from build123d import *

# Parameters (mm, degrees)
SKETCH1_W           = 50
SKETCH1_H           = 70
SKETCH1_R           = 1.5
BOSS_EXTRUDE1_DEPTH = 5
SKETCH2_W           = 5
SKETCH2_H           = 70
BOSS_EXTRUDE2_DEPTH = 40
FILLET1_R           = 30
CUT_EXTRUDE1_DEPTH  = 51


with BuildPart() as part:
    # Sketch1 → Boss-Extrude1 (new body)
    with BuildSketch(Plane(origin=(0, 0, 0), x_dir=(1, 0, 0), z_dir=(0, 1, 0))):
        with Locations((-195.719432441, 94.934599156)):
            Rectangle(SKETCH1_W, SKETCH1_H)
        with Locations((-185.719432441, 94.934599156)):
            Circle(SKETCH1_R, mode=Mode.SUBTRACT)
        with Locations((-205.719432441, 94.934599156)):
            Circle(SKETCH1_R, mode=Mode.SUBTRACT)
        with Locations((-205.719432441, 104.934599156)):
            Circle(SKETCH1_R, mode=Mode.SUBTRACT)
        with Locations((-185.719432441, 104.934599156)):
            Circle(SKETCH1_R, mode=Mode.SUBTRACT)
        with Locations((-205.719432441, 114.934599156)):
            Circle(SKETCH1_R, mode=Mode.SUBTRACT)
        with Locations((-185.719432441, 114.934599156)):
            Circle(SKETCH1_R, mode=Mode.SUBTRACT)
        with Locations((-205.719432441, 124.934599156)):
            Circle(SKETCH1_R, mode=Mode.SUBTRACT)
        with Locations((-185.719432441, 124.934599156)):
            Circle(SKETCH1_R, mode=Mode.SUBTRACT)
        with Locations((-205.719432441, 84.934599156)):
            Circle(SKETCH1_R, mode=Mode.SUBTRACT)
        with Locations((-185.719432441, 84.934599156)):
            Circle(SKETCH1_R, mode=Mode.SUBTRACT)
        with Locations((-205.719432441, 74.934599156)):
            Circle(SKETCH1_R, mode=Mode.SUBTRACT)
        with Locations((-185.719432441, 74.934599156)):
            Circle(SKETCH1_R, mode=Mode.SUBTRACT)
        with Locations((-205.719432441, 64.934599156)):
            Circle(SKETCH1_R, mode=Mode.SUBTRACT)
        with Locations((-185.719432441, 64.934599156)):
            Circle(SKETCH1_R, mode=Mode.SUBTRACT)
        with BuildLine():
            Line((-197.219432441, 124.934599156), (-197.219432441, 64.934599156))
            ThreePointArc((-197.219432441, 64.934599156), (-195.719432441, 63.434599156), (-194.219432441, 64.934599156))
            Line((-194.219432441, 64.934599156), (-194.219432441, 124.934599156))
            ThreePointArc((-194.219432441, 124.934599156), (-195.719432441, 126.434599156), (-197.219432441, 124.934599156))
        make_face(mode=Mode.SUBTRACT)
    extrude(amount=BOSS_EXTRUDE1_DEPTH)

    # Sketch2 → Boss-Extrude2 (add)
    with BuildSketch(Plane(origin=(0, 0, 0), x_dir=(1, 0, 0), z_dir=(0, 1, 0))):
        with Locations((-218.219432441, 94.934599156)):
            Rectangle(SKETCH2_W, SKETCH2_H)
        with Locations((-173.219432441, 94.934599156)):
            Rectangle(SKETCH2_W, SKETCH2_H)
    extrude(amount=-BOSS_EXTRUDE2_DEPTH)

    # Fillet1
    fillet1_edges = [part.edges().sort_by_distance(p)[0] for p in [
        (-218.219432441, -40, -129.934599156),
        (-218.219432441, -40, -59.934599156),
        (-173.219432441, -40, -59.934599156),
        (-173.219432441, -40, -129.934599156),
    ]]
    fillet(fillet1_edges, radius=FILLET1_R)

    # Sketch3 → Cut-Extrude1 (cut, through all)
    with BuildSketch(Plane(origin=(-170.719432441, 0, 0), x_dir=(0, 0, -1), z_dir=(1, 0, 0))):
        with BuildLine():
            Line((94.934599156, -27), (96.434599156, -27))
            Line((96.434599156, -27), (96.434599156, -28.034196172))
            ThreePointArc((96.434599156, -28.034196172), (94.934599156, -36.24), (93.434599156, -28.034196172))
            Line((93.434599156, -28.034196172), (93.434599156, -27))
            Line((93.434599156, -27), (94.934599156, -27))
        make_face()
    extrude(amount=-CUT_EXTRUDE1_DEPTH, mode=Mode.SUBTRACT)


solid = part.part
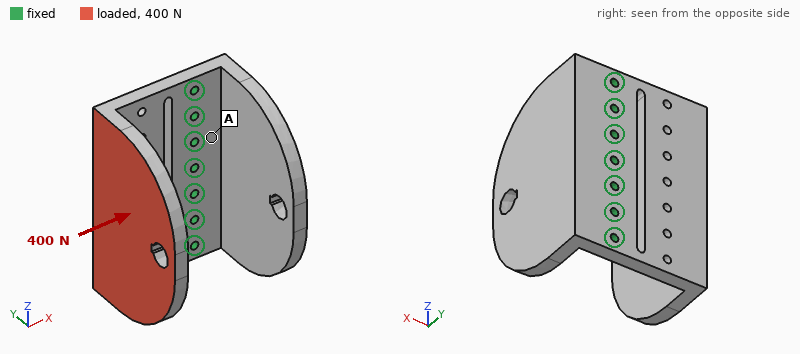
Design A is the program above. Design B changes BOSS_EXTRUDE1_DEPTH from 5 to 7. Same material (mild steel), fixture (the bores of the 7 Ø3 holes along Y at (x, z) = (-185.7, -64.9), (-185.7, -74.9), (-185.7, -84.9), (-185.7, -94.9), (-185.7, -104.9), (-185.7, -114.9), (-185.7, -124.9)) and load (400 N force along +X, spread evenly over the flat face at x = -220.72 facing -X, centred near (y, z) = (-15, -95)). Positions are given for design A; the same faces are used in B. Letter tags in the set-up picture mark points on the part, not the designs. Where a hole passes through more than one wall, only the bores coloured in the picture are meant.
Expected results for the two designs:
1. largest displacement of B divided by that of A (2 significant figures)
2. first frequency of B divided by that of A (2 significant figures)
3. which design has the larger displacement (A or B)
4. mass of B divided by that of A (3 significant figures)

0.42
1.5
A
1.16
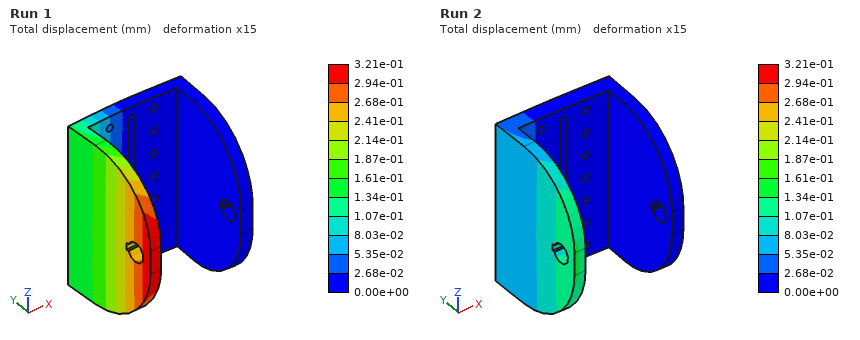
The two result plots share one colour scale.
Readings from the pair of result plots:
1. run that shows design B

Run 2
